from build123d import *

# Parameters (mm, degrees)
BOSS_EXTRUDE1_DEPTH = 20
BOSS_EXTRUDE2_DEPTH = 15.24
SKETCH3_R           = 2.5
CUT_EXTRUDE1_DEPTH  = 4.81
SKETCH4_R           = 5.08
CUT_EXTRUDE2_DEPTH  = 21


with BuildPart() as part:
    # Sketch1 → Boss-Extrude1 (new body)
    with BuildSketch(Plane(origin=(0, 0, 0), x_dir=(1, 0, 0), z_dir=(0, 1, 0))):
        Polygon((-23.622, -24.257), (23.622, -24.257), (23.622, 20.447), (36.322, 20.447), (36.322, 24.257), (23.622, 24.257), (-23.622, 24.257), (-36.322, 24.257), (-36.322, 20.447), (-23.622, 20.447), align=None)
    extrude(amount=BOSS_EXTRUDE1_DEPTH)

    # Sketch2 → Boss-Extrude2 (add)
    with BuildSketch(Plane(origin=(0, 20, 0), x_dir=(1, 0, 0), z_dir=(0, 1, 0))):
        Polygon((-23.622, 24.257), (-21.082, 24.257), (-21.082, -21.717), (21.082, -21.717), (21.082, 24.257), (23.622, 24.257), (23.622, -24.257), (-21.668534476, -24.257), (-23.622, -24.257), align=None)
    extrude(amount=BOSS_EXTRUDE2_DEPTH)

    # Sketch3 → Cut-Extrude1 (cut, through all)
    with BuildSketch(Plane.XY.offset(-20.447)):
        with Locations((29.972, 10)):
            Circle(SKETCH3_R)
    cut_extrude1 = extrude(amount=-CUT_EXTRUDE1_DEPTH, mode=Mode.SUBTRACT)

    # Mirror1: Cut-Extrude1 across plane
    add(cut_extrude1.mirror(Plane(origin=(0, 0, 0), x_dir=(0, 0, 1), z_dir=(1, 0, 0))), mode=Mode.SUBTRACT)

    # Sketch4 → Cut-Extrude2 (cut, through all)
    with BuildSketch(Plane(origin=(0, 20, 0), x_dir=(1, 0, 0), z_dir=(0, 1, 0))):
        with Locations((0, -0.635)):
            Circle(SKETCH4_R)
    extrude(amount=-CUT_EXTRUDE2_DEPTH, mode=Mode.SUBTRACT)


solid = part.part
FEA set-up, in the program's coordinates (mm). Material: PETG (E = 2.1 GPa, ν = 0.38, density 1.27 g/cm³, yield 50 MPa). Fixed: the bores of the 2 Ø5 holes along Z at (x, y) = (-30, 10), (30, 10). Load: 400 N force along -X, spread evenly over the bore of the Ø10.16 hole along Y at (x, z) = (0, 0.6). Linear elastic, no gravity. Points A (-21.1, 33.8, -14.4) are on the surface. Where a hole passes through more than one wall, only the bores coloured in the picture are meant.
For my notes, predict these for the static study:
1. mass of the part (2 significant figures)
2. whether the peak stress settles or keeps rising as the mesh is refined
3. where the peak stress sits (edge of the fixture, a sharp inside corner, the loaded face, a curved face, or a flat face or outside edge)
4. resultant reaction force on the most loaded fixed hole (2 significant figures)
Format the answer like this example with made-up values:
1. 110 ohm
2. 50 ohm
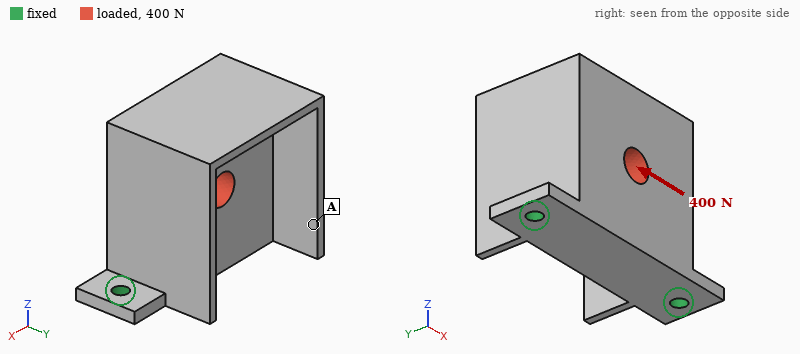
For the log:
1. 65 g
2. keeps rising
3. edge of the fixture
4. 270 N
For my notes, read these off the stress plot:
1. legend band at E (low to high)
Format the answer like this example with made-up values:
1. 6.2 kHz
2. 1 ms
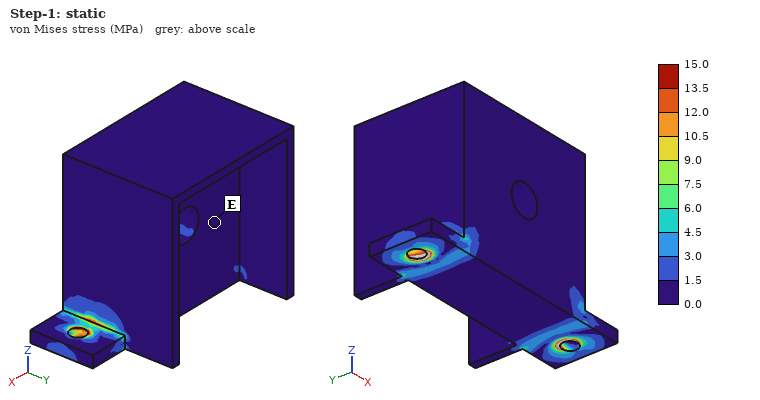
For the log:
1. 0.0 to 1.5 MPa
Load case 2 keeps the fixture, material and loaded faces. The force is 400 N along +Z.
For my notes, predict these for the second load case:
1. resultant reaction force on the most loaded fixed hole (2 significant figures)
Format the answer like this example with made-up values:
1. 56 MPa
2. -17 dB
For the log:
1. 230 N
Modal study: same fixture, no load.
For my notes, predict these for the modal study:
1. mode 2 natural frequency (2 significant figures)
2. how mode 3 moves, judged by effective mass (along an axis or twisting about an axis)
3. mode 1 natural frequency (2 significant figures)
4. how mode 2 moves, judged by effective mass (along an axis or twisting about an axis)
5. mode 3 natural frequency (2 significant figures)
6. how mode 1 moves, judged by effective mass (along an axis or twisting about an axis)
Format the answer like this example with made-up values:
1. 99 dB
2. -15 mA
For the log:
1. 1100 Hz
2. along Z
3. 230 Hz
4. along X
5. 1400 Hz
6. along Y
